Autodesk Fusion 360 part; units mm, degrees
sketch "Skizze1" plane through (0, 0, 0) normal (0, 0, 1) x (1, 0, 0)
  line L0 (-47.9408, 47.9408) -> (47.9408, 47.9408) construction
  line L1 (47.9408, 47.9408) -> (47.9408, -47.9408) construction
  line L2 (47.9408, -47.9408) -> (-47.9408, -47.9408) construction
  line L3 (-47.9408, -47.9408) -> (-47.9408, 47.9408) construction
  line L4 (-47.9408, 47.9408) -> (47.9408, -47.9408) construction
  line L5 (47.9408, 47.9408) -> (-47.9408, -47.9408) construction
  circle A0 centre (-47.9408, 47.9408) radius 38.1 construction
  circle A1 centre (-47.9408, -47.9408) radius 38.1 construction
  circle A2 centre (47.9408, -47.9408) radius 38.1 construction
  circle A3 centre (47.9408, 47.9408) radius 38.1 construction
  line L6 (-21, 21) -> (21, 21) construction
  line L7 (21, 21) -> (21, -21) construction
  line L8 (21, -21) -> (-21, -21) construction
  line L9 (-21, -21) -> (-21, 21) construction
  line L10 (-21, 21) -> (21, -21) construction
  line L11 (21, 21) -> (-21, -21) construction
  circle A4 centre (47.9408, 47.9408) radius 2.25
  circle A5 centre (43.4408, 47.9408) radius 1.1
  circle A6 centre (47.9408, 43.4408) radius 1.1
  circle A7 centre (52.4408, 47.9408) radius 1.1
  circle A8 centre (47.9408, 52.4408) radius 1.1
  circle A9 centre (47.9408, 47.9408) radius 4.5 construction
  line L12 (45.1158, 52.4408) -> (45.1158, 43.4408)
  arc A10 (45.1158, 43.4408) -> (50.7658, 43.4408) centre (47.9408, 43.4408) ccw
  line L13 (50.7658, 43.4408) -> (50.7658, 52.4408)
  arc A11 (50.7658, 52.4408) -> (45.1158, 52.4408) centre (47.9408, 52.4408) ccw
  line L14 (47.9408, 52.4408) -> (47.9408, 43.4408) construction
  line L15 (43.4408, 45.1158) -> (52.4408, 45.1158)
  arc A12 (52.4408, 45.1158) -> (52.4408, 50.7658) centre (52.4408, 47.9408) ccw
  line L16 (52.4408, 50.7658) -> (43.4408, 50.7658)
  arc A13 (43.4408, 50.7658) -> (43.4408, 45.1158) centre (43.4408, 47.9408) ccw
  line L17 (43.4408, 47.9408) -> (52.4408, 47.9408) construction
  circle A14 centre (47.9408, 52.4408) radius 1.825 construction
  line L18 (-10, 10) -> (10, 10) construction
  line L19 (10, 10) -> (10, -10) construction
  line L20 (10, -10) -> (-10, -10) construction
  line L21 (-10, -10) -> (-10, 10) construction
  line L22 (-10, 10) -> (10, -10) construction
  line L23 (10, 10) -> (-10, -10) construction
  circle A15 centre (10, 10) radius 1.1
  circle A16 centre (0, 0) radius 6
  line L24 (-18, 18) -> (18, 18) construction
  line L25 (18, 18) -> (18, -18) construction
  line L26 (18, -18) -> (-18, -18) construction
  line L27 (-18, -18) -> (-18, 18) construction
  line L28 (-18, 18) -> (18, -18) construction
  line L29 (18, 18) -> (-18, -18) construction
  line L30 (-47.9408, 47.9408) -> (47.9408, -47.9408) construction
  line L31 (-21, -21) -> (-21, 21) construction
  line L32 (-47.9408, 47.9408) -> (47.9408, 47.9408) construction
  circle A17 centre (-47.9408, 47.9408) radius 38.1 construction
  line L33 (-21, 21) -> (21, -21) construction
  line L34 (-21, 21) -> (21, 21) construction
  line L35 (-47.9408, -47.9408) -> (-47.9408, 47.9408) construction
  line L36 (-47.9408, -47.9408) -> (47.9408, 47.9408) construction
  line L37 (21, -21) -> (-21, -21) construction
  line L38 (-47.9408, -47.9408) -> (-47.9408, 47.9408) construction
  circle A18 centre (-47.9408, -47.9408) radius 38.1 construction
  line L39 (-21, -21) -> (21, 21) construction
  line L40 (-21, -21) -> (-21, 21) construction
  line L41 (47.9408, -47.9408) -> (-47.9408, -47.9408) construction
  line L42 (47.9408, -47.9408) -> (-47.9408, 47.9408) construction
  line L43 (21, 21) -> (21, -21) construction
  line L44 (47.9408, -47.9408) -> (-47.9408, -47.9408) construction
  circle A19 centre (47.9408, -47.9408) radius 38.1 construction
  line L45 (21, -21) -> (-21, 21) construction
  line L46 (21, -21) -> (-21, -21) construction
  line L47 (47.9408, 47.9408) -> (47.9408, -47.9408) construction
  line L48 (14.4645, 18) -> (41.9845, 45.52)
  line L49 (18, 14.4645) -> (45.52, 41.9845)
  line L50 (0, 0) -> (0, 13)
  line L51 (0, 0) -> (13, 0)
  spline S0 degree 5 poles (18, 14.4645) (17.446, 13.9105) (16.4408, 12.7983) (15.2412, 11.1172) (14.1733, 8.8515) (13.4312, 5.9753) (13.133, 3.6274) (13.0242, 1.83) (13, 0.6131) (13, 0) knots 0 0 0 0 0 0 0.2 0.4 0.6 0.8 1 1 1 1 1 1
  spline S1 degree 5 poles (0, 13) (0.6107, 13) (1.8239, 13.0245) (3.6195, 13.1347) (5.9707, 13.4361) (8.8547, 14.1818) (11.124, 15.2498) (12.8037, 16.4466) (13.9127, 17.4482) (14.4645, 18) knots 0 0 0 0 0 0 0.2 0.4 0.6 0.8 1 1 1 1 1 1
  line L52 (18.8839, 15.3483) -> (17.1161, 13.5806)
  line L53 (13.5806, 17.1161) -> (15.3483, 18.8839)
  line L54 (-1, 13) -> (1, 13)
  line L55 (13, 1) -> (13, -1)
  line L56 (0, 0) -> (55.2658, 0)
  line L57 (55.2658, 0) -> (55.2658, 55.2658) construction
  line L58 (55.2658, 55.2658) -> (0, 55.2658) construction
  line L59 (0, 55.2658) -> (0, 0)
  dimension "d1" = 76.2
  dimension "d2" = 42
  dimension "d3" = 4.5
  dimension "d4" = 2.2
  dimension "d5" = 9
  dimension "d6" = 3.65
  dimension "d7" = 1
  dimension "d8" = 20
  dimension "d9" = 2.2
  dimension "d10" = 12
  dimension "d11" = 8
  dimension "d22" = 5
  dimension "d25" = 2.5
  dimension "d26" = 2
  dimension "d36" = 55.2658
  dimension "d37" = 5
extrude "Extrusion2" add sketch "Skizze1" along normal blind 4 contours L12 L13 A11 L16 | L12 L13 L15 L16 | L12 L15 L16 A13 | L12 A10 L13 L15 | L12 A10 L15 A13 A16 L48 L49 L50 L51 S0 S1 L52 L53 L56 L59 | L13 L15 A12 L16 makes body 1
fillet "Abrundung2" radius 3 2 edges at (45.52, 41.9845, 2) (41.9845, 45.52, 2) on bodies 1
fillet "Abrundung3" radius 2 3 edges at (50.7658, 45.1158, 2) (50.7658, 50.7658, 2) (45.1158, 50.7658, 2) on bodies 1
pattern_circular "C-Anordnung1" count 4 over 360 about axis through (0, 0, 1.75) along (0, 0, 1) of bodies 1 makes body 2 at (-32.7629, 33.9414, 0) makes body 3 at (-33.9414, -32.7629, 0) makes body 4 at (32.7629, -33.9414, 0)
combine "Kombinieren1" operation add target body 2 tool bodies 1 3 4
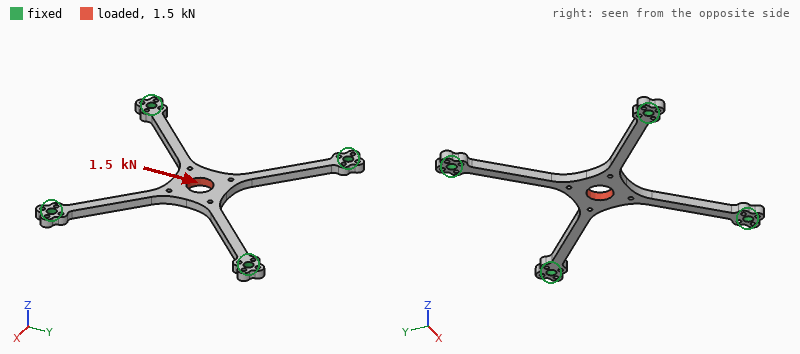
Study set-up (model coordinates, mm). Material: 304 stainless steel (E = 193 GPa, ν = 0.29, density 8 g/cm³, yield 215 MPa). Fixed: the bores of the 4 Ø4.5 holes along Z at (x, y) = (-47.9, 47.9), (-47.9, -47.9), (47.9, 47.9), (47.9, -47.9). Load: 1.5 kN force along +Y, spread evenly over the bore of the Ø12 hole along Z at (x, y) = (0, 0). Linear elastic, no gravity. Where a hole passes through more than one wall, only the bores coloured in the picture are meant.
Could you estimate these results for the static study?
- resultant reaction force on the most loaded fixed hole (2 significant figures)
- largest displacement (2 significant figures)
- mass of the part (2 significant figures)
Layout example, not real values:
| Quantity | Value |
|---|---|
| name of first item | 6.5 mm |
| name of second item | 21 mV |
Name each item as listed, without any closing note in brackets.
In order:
| Quantity | Value |
|---|---|
| resultant reaction force on the most loaded fixed hole | 520 N |
| largest displacement | 11 µm |
| mass of the part | 60 g |
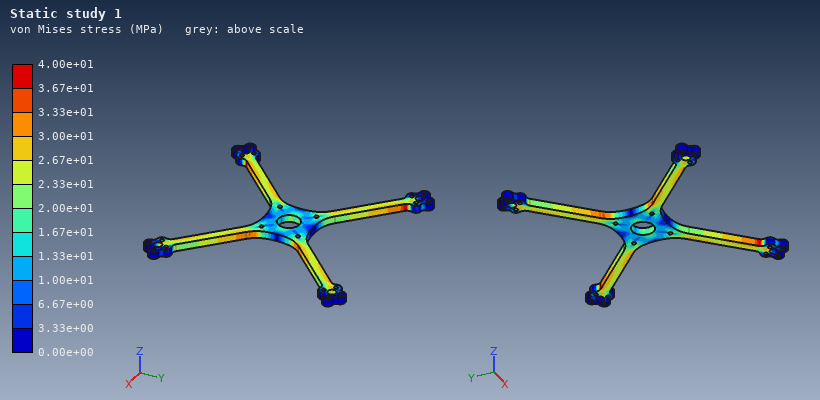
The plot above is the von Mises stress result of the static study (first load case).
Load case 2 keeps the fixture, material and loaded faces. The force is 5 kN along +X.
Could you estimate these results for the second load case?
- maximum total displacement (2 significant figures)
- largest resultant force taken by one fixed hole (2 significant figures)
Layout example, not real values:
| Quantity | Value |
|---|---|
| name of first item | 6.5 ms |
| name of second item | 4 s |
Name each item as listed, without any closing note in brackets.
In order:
| Quantity | Value |
|---|---|
| maximum total displacement | 36 µm |
| largest resultant force taken by one fixed hole | 1.7 kN |
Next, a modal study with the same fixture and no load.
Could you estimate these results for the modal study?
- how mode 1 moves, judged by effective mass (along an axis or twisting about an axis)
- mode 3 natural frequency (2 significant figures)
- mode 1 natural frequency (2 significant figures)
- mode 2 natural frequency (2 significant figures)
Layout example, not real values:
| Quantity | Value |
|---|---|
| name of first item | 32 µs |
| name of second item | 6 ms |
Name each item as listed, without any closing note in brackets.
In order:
| Quantity | Value |
|---|---|
| how mode 1 moves, judged by effective mass | along Z |
| mode 3 natural frequency | 3200 Hz |
| mode 1 natural frequency | 1100 Hz |
| mode 2 natural frequency | 3200 Hz |
